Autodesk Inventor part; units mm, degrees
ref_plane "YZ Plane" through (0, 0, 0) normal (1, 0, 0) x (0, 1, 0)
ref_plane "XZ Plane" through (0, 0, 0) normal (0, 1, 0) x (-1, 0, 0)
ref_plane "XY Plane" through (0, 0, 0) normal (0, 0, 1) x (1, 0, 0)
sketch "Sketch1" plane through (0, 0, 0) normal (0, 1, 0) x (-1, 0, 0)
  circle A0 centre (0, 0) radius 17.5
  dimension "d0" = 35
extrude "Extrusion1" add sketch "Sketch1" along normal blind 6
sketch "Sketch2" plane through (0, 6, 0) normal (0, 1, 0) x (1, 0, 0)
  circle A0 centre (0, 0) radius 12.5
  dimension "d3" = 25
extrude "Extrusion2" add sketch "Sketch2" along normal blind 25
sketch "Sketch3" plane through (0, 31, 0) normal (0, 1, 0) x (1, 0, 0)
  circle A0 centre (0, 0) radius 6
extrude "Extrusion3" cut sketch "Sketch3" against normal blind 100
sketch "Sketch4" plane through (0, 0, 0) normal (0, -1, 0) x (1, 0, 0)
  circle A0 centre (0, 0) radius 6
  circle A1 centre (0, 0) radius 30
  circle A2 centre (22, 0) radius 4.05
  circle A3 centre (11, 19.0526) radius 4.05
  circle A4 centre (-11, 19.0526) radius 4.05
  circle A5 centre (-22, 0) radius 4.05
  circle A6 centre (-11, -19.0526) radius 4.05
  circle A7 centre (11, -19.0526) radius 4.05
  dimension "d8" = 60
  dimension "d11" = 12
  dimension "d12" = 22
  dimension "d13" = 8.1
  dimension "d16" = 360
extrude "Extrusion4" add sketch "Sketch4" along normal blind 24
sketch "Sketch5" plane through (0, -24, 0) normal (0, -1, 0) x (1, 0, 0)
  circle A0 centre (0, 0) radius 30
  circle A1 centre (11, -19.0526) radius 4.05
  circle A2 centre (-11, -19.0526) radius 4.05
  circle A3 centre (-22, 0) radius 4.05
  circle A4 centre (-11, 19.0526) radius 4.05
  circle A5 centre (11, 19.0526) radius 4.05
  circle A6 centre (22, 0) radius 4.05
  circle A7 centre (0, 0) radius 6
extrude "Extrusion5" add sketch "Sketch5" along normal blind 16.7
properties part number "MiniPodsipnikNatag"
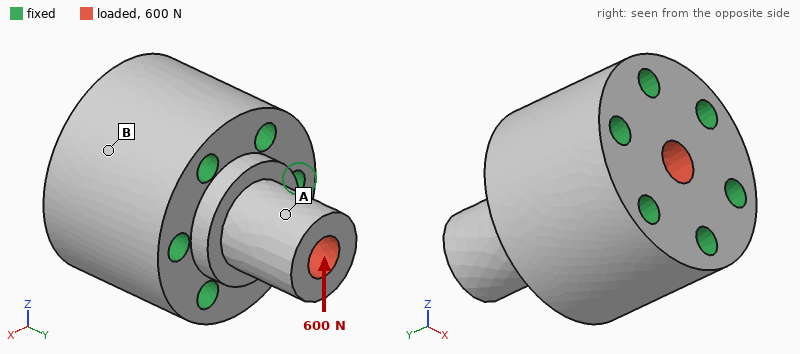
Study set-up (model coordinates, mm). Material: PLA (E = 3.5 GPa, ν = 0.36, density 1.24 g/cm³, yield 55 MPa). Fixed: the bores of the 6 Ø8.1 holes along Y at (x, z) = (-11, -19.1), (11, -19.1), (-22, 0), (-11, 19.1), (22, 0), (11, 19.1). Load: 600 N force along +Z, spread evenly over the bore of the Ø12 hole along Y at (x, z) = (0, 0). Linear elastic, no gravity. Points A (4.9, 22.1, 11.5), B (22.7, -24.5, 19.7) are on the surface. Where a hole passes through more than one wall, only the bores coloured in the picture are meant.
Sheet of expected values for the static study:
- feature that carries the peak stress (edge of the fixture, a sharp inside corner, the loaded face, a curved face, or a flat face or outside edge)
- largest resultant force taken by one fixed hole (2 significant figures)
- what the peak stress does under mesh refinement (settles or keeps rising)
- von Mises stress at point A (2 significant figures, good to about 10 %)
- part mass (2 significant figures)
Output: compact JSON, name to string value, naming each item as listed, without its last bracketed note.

{"feature that carries the peak stress": "edge of the fixture", "largest resultant force taken by one fixed hole": "180 N", "what the peak stress does under mesh refinement": "keeps rising", "von Mises stress at point A": "0.36 MPa", "part mass": "140 g"}
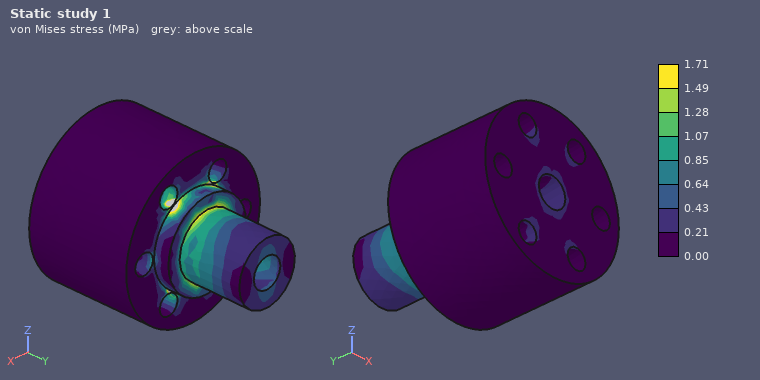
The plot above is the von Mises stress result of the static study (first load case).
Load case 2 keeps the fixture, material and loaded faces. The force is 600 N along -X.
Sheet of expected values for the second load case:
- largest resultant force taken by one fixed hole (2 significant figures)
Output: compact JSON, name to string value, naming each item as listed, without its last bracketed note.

{"largest resultant force taken by one fixed hole": "200 N"}
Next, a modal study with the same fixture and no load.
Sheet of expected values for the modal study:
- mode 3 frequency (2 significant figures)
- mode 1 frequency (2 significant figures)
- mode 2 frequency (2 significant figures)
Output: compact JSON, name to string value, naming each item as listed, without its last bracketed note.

{"mode 3 frequency": "8700 Hz", "mode 1 frequency": "5100 Hz", "mode 2 frequency": "5100 Hz"}
